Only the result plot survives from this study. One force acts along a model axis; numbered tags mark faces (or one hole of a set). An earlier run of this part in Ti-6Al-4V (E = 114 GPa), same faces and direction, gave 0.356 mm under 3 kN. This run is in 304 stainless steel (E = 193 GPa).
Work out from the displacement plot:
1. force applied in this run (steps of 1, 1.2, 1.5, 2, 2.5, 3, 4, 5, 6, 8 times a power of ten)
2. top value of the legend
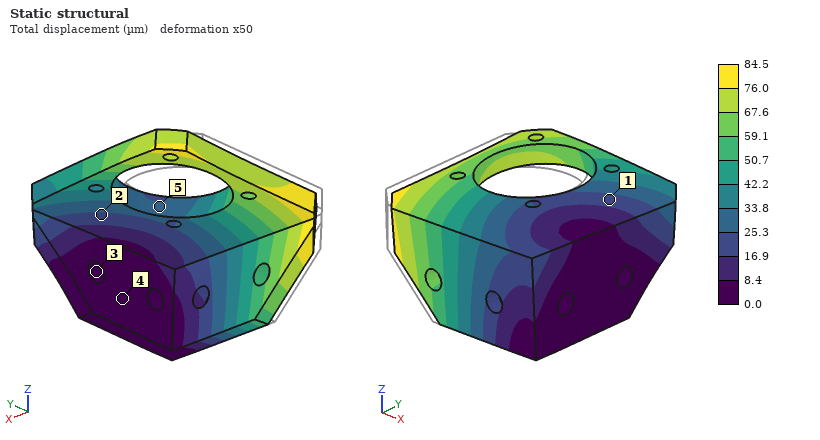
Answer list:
1.2 kN
84.5 µm
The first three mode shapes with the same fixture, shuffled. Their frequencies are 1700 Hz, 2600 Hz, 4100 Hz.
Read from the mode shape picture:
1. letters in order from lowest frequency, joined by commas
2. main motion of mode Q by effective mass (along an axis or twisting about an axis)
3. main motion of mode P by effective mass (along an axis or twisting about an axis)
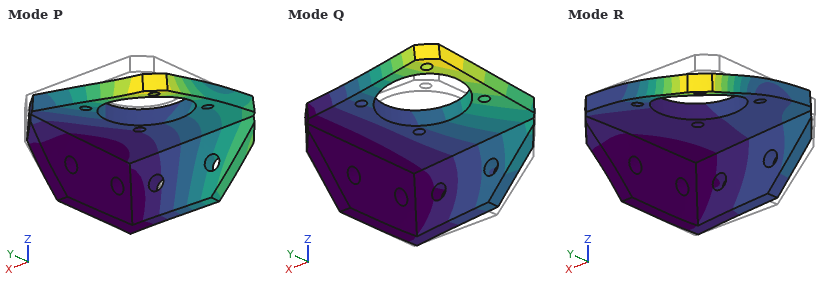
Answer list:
Q, P, R
along Z
along Y
